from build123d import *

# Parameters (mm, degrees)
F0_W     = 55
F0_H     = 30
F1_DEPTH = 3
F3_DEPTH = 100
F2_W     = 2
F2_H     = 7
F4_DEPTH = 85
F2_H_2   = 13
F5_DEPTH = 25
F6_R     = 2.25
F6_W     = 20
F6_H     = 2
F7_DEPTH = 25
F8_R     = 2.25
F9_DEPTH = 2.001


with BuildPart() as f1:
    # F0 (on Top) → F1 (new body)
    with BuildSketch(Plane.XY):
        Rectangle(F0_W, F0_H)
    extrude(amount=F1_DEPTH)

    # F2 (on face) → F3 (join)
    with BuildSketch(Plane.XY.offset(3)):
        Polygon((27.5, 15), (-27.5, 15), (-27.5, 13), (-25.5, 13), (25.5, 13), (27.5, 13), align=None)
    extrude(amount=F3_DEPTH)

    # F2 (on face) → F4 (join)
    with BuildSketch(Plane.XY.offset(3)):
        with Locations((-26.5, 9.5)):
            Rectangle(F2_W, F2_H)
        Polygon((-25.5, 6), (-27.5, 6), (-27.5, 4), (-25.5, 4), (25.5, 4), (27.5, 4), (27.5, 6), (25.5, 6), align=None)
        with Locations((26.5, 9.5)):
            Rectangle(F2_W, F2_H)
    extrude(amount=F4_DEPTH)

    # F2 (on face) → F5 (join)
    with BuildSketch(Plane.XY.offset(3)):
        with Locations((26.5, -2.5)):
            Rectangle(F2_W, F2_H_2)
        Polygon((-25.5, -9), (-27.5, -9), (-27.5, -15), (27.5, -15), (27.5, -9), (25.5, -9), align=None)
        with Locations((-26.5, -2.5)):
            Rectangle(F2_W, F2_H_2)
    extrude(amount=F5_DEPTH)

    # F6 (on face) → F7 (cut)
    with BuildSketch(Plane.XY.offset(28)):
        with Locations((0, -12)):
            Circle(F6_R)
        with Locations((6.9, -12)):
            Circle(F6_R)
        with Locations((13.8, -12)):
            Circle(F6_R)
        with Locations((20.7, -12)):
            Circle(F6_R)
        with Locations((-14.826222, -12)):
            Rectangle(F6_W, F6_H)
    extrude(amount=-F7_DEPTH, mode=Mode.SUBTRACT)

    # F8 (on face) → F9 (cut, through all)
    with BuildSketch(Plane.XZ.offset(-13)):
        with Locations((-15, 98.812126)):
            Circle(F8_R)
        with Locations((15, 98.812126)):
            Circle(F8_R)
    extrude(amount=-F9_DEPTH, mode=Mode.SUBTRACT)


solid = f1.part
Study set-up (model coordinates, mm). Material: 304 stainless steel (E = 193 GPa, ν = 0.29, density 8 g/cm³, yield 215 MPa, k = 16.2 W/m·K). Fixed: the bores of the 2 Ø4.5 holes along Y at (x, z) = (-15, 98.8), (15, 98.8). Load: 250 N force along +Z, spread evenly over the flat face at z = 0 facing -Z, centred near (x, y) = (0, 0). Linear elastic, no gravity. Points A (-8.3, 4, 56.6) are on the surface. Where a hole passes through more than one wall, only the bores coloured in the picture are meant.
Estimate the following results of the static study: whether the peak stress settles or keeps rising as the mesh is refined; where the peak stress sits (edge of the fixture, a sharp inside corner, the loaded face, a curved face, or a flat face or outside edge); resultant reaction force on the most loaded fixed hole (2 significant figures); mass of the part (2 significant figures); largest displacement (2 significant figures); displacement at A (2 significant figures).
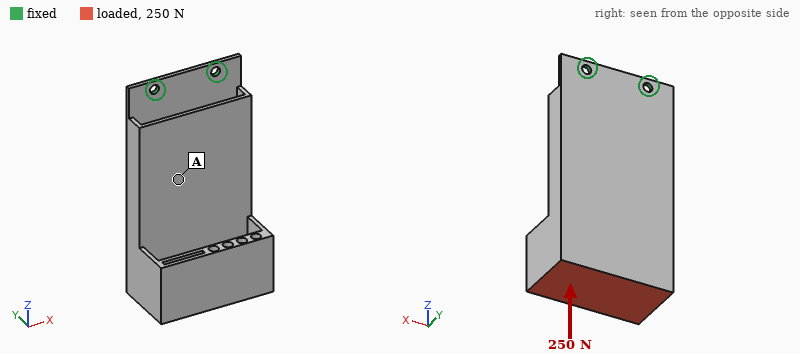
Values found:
keeps rising
edge of the fixture
140 N
280 g
0.80 mm
0.29 mm
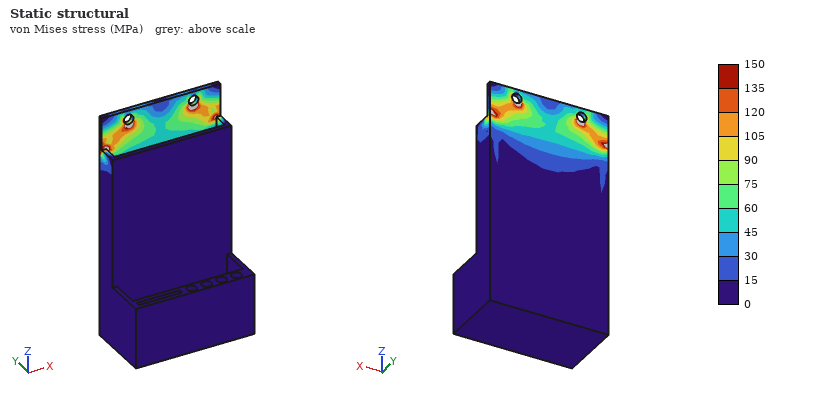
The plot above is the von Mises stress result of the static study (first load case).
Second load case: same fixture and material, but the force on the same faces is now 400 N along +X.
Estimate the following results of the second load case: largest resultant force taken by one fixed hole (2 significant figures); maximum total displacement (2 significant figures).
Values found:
1.2 kN
0.12 mm
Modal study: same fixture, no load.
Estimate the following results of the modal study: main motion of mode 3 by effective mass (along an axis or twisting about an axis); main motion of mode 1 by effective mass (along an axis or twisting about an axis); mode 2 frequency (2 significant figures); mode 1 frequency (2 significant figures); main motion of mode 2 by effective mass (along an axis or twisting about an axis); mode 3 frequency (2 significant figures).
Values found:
along X
along Y
640 Hz
97 Hz
along X
1600 Hz
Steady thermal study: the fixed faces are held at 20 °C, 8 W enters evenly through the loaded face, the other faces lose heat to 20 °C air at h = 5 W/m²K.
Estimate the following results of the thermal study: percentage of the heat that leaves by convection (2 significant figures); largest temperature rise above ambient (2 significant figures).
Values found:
85 %
76 K
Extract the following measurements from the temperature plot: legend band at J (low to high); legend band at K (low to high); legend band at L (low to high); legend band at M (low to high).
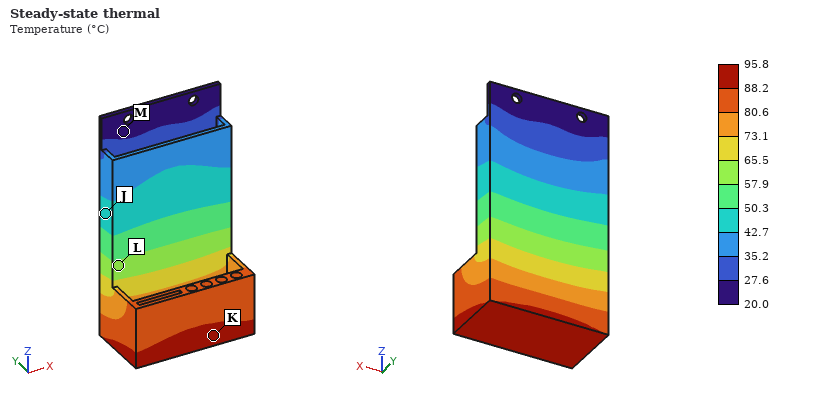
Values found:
42.7 to 50.3 °C
88.2 to 95.8 °C
57.9 to 65.5 °C
20.0 to 27.6 °C
